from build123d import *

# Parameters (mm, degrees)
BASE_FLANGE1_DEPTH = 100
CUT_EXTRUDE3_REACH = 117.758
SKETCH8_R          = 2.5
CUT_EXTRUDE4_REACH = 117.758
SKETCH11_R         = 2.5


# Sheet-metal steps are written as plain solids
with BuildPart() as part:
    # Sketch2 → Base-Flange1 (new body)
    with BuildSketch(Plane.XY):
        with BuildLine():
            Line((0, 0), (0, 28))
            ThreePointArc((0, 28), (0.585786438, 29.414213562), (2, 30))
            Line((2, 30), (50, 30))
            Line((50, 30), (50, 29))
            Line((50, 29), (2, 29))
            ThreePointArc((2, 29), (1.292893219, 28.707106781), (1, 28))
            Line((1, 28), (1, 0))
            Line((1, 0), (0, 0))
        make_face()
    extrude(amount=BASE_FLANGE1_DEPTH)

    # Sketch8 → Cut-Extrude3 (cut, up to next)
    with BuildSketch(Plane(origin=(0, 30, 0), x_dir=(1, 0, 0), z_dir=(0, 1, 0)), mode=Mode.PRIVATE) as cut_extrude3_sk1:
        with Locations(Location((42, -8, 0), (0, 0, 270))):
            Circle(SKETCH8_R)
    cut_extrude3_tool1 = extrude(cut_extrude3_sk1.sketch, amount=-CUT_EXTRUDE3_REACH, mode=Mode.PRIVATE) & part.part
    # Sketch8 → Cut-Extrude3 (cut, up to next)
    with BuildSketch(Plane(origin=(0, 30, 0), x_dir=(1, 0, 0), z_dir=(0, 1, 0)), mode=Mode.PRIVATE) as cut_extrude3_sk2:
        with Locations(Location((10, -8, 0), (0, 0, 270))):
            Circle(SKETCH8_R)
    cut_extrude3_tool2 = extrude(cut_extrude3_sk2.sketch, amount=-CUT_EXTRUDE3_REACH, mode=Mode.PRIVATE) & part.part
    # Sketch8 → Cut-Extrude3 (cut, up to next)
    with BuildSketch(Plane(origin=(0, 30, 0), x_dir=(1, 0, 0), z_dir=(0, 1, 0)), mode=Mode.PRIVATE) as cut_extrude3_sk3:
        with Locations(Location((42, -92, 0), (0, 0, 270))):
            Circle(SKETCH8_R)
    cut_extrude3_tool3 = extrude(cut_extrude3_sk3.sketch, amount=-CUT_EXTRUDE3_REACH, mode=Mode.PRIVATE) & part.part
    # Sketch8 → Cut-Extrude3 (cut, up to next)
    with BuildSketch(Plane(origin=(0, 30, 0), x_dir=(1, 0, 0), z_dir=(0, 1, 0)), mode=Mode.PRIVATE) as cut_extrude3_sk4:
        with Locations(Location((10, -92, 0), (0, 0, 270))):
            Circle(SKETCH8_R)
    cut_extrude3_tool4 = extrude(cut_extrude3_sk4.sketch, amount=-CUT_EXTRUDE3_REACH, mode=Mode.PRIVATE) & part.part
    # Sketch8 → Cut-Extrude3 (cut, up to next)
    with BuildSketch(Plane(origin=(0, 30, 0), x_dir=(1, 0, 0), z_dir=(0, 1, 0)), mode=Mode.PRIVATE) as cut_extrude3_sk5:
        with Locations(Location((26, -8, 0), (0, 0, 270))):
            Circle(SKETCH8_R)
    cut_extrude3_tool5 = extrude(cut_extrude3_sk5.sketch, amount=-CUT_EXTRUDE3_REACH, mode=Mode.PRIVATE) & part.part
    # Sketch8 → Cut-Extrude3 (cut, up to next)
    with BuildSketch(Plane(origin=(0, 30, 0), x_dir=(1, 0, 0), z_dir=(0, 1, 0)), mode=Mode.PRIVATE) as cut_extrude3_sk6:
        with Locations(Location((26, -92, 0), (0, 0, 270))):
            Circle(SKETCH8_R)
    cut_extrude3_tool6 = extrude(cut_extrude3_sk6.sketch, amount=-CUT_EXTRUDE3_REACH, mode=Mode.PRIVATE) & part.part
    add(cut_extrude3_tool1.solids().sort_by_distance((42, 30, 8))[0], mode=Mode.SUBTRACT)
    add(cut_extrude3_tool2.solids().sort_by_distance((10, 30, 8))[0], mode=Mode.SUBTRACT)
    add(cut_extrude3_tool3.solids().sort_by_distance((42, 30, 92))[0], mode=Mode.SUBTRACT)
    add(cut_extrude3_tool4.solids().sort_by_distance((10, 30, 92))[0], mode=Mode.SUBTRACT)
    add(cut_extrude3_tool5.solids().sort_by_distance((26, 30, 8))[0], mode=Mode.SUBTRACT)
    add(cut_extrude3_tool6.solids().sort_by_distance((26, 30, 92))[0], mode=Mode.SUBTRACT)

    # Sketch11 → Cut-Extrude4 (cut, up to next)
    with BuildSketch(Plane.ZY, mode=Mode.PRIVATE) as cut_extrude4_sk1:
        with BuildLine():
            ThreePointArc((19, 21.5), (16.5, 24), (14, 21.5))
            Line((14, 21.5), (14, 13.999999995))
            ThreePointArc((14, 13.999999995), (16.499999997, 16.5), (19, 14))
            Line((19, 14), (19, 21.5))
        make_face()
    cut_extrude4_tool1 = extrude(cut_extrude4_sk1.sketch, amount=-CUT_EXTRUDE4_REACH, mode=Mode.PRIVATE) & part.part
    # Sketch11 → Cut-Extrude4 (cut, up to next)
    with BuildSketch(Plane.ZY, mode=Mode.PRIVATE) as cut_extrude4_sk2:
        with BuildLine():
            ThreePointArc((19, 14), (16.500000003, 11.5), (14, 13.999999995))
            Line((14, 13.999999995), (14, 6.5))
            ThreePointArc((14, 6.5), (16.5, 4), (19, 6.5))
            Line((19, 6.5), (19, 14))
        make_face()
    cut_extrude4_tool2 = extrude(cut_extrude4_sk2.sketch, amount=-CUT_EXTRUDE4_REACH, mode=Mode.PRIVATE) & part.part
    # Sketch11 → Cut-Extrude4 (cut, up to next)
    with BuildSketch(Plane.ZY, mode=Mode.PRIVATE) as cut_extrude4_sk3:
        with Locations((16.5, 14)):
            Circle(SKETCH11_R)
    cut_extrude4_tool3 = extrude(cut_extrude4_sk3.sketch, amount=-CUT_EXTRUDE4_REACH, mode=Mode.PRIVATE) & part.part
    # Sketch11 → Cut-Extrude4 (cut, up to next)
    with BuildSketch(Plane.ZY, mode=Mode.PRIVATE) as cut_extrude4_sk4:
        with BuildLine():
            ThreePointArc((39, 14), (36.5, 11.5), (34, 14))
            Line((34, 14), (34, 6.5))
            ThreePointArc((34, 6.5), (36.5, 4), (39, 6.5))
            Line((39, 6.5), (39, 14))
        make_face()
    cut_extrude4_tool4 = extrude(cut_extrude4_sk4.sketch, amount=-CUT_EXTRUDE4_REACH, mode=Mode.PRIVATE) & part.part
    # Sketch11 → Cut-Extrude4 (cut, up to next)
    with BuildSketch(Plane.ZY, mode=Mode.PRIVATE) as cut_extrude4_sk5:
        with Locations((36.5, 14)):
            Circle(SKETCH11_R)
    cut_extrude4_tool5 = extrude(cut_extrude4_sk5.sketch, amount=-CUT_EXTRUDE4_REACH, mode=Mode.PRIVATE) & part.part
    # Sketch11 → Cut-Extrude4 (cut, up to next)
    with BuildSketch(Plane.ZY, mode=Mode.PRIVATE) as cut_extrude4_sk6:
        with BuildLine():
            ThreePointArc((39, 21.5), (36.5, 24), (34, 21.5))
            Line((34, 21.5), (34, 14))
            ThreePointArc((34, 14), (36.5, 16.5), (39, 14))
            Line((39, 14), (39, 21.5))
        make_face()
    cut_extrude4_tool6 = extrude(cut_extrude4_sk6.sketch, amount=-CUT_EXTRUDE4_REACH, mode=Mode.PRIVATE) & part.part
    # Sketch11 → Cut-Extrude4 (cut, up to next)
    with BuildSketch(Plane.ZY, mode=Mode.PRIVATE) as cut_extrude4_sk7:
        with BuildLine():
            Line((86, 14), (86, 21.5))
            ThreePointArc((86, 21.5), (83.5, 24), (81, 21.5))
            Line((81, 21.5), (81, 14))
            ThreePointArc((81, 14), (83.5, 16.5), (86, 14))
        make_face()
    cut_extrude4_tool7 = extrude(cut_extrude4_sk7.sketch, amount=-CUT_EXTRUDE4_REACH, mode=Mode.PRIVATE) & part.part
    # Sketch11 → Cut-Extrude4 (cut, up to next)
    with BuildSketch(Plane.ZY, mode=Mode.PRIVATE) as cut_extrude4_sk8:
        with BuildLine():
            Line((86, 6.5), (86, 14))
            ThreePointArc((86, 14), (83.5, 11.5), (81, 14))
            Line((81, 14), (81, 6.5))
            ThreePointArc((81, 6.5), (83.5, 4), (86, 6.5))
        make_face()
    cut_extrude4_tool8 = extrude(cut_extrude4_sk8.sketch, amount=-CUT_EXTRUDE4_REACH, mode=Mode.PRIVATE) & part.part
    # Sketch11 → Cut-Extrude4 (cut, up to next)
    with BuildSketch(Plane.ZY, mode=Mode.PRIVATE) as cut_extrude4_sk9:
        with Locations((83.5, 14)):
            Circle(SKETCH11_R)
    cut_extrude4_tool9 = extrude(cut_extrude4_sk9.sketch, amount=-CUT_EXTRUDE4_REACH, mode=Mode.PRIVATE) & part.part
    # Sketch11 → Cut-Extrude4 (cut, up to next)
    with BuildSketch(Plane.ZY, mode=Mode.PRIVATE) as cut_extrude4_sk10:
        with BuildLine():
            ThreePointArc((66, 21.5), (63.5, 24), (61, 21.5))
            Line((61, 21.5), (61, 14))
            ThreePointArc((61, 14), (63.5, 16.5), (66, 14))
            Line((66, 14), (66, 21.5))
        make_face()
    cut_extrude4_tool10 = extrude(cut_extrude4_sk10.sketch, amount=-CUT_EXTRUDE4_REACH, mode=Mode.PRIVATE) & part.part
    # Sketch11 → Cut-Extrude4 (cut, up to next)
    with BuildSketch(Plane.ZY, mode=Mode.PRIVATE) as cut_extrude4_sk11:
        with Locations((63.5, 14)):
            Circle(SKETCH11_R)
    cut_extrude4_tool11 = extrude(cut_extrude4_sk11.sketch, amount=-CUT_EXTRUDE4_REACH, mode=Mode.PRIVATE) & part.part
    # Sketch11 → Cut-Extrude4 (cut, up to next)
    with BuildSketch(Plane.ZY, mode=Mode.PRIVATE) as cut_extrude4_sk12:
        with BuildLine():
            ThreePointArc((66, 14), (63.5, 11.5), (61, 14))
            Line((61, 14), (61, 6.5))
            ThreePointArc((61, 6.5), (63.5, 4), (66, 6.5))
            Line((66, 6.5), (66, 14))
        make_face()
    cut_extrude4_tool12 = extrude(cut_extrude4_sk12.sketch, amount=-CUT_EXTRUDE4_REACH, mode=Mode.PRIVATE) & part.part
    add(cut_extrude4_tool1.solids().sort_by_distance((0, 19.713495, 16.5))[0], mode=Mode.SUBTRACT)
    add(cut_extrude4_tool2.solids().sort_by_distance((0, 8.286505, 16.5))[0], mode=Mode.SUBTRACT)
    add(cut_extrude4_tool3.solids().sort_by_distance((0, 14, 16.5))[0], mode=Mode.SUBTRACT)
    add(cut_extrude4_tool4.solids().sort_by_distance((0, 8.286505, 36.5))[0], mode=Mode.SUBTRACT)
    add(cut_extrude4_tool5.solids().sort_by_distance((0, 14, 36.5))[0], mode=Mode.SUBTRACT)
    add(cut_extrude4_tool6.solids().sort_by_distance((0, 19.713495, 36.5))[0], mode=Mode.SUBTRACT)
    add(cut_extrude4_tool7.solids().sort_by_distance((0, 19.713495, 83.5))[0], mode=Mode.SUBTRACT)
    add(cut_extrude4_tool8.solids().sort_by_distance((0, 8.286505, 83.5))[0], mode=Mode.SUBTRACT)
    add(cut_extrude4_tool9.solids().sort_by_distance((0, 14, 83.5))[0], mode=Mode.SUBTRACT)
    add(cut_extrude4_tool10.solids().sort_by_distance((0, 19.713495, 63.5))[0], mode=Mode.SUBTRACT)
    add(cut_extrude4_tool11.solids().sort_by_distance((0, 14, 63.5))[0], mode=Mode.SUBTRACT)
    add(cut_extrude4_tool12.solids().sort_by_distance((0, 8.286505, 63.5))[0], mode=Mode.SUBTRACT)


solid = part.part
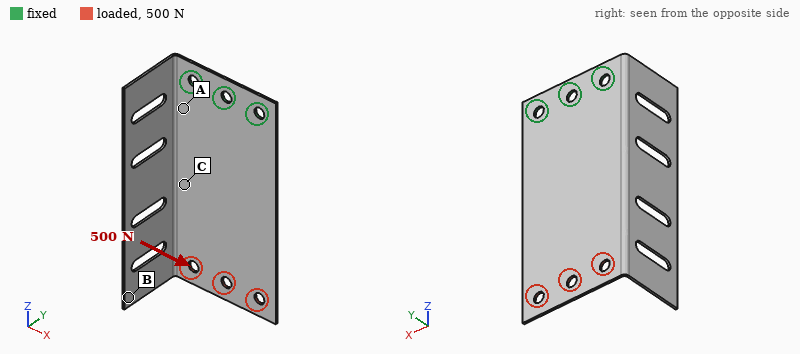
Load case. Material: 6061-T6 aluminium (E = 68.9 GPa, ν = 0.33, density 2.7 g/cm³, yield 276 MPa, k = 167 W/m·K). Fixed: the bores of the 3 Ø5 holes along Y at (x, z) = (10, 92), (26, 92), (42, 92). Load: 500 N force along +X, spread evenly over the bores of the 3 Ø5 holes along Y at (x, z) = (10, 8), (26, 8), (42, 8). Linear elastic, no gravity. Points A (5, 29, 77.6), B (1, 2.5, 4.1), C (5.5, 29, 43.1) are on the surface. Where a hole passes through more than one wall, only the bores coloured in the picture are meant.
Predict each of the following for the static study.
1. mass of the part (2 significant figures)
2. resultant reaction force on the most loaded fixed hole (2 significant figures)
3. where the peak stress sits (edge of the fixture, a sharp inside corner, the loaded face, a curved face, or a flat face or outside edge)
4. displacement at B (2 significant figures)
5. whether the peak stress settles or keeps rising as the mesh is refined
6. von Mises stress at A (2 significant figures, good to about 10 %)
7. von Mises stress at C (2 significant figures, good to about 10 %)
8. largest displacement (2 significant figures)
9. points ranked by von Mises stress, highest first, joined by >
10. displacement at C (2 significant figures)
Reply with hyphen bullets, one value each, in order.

- 20 g
- 1.2 kN
- edge of the fixture
- 0.21 mm
- keeps rising
- 51 MPa
- 27 MPa
- 0.24 mm
- A > C > B
- 0.10 mm
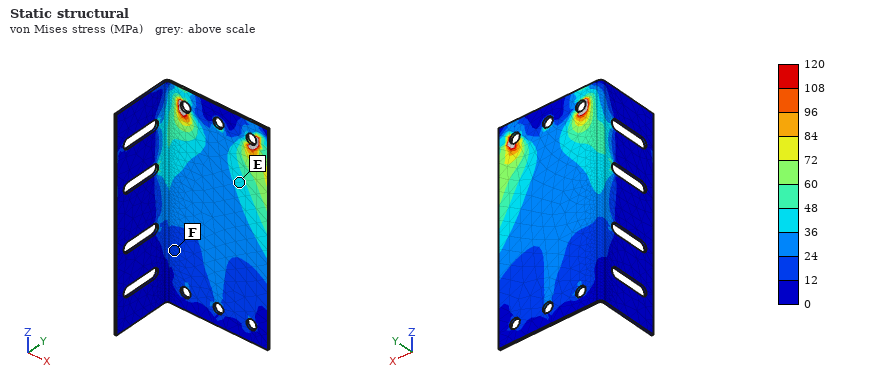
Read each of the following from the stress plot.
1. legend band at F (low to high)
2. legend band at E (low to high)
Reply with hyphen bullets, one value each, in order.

- 12 to 24 MPa
- 36 to 48 MPa
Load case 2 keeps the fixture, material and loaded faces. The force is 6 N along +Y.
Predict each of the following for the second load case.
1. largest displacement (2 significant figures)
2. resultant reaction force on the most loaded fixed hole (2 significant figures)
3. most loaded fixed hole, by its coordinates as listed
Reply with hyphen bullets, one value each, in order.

- 1.4 mm
- 4.9 N
- (26, 92)
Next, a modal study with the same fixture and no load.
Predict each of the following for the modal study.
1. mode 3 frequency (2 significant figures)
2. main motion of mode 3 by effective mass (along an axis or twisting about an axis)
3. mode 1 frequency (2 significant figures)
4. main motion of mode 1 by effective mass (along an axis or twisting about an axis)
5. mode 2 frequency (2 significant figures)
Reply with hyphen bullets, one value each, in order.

- 700 Hz
- along X
- 160 Hz
- along Y
- 280 Hz
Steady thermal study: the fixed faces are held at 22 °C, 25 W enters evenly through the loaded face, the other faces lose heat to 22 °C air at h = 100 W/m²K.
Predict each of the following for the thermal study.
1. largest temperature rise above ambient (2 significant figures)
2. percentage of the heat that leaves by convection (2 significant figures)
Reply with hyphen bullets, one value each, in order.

- 70 K
- 93 %
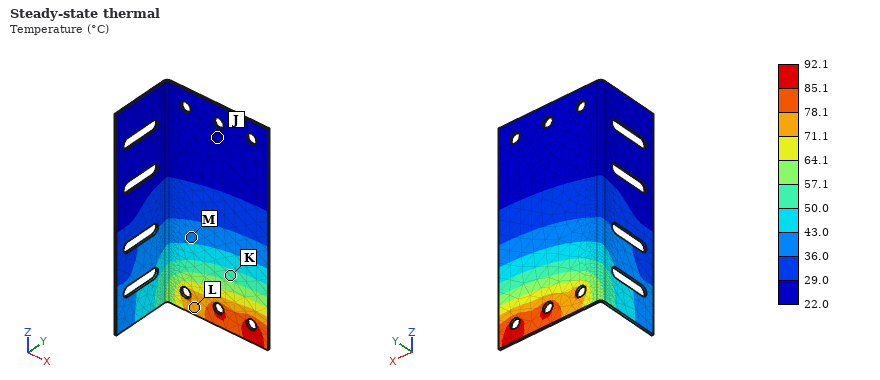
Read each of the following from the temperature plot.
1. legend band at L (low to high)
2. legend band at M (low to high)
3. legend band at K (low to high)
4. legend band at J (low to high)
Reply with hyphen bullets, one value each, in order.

- 71.1 to 78.1 °C
- 36.0 to 43.0 °C
- 50.0 to 57.1 °C
- 22.0 to 29.0 °C
